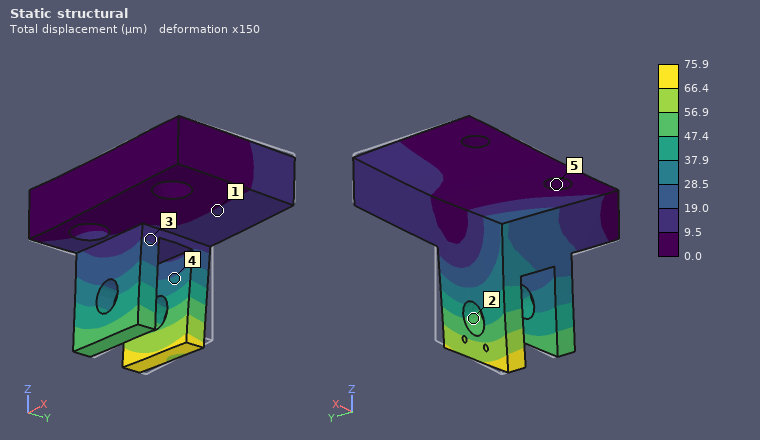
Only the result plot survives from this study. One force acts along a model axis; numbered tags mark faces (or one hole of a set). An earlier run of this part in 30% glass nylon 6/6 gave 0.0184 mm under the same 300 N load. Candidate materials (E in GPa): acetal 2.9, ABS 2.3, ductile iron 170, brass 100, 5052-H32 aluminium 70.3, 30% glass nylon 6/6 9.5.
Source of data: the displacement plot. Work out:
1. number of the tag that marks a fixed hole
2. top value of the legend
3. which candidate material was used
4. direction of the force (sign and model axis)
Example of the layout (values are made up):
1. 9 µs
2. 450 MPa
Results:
1. 5
2. 75.9 µm
3. ABS
4. -X
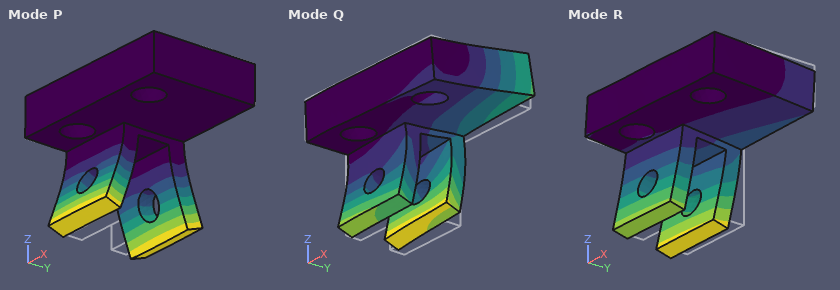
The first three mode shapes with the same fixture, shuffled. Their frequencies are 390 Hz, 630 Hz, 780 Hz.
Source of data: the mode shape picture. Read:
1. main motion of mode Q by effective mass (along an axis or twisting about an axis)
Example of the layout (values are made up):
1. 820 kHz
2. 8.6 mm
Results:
1. along Z
